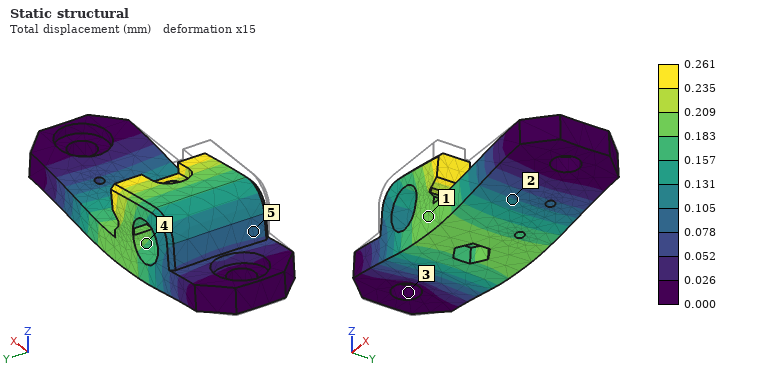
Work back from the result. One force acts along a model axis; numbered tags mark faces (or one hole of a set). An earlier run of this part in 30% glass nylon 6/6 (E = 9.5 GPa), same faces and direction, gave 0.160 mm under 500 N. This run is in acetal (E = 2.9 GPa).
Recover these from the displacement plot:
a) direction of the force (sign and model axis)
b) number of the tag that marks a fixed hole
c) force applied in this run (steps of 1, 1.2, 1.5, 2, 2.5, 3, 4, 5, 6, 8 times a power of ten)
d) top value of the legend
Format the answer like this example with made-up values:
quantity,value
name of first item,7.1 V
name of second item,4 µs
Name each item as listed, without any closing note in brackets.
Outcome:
quantity,value
direction of the force,-Z
number of the tag that marks a fixed hole,3
force applied in this run,250 N
top value of the legend,0.261 mm
